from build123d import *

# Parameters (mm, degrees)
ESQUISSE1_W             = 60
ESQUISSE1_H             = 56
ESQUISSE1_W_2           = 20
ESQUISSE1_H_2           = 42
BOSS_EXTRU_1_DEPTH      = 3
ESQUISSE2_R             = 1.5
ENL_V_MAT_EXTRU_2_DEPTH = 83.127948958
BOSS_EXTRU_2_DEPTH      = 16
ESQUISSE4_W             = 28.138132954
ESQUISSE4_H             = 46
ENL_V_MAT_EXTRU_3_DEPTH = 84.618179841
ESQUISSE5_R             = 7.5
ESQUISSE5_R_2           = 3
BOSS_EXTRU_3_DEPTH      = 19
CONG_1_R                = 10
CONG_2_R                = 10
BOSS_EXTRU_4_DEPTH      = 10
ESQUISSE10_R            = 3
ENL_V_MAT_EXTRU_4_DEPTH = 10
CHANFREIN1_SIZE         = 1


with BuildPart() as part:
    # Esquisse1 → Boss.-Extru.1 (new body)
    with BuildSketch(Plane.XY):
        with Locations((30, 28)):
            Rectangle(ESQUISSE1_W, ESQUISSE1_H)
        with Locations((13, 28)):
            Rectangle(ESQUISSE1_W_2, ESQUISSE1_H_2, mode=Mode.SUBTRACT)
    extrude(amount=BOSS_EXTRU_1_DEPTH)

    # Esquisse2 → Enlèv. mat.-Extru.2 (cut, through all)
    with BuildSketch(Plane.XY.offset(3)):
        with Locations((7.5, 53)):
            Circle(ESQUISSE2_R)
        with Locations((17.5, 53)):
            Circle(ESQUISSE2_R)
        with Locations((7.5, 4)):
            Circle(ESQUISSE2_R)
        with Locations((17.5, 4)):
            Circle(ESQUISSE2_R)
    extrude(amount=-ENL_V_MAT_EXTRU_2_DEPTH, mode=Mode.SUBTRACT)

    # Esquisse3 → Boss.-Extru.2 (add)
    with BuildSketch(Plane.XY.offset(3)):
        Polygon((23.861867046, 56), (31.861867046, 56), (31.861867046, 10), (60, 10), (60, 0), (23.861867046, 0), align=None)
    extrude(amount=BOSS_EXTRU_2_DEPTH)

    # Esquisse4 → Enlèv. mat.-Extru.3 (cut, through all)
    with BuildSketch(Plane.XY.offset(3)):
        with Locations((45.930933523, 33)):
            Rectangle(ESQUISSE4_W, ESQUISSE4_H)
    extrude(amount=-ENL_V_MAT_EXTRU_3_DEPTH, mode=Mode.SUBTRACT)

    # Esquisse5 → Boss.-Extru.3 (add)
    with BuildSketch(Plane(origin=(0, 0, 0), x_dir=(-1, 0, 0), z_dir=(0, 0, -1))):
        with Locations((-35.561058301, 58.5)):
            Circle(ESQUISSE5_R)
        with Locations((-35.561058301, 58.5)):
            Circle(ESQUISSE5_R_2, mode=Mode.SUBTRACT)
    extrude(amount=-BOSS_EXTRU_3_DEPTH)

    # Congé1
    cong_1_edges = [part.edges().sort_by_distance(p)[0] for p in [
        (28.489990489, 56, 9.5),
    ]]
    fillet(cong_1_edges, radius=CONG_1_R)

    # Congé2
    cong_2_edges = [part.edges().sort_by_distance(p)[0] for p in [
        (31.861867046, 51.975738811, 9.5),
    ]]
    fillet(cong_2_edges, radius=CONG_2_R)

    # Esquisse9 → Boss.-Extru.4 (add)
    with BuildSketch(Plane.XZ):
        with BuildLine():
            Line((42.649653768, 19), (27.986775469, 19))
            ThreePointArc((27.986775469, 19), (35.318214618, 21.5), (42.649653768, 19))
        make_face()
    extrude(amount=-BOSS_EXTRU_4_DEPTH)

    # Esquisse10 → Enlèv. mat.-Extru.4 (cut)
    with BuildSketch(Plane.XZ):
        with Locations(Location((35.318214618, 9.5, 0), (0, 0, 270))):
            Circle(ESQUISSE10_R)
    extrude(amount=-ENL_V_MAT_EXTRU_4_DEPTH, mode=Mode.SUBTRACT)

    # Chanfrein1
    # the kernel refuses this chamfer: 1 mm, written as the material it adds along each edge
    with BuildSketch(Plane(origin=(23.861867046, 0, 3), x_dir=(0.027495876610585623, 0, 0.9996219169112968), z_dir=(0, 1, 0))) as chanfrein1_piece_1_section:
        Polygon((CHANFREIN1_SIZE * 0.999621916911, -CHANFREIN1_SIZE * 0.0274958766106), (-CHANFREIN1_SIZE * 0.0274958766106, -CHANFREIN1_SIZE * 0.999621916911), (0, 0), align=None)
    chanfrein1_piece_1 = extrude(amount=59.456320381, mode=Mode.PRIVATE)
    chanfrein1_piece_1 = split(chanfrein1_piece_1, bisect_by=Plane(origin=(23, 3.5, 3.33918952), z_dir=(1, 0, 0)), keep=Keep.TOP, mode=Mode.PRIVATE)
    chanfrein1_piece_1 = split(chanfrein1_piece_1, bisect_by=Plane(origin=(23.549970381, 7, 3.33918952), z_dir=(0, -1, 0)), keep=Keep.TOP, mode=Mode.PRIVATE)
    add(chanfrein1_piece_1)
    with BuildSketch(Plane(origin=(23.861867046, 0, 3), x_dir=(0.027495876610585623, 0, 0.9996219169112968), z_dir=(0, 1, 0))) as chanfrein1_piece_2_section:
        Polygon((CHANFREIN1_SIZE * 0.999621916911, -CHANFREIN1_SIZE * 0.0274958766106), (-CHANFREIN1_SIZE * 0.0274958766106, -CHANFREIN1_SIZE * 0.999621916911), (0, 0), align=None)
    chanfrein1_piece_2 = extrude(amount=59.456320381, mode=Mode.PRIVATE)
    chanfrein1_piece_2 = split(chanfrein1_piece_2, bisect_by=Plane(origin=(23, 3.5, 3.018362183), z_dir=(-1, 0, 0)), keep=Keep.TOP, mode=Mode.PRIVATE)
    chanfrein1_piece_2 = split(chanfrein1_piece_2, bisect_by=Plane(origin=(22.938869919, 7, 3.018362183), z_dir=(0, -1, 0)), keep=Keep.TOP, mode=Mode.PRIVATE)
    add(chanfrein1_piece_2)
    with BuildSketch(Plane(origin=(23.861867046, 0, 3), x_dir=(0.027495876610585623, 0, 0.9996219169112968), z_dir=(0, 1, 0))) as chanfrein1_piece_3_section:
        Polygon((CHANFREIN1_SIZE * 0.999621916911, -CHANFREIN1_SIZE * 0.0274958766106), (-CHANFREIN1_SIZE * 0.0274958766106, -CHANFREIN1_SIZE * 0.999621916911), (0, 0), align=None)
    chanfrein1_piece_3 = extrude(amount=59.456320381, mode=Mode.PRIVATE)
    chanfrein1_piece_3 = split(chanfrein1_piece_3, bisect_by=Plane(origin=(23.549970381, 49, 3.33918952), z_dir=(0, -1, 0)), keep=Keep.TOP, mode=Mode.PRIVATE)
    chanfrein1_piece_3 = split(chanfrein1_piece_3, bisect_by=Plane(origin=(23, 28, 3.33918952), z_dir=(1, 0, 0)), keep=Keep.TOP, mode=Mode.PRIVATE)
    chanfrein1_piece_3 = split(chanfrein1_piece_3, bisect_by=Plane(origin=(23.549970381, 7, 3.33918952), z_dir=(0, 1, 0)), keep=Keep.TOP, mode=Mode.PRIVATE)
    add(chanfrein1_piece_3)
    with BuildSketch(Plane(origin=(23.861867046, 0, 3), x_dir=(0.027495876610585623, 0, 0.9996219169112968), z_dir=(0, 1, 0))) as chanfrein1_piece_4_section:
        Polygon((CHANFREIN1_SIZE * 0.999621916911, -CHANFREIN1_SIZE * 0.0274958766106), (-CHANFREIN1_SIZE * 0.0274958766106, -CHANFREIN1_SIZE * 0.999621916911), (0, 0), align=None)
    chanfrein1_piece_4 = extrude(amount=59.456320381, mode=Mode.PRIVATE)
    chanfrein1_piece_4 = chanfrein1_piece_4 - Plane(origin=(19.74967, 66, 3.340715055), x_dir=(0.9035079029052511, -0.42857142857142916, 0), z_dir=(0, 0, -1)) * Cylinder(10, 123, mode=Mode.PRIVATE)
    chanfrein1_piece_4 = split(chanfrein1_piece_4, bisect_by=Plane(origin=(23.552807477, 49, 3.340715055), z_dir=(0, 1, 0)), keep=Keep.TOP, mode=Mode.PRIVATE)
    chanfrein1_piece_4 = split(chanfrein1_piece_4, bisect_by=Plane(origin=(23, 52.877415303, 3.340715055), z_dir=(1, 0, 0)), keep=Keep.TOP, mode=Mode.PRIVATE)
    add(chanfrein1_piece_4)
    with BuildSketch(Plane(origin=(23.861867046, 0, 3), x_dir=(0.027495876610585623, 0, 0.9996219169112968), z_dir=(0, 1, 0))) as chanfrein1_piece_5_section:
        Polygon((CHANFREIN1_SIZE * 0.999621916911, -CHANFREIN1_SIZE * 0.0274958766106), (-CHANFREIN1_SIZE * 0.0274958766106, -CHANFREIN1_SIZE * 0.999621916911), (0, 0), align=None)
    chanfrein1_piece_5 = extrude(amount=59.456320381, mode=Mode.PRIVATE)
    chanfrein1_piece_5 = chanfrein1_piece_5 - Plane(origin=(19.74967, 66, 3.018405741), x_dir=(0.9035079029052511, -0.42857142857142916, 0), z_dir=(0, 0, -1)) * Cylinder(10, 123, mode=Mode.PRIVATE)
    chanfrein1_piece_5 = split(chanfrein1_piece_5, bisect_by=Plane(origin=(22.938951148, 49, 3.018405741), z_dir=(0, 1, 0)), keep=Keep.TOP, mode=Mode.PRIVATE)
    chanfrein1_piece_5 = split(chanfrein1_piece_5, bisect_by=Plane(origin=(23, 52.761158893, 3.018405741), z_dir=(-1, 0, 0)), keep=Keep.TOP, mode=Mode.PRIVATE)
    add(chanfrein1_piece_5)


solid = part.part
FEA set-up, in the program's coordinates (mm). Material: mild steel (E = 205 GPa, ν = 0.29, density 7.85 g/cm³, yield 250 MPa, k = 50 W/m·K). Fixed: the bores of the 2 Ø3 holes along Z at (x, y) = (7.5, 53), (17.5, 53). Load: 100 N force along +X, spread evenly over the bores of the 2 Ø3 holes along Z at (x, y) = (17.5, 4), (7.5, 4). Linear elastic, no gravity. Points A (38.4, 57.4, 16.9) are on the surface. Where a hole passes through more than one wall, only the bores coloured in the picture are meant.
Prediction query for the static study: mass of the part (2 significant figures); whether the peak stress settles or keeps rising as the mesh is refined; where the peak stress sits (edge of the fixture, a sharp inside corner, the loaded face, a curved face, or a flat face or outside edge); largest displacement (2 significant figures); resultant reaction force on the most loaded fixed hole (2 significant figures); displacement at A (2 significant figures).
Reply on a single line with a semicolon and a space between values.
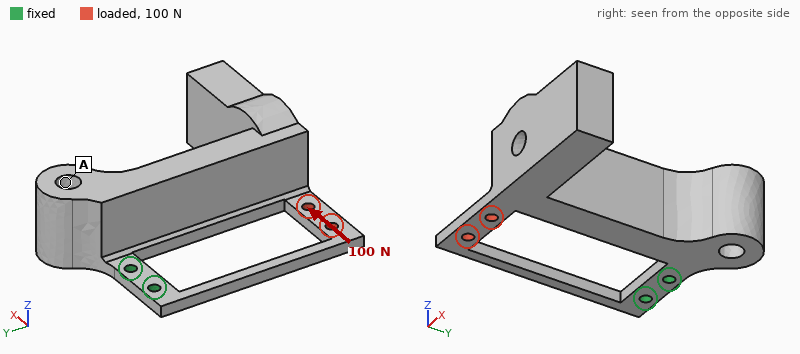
140 g; keeps rising; a sharp inside corner; 96 µm; 220 N; 23 µm
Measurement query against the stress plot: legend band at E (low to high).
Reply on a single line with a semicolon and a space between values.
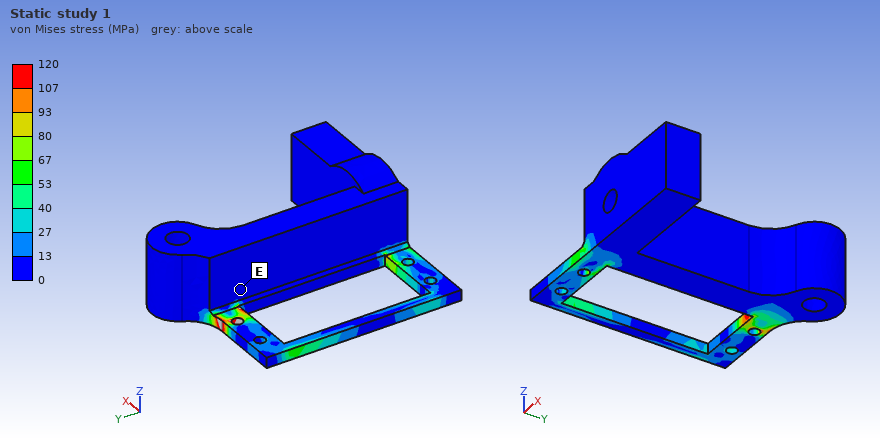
0 to 13 MPa
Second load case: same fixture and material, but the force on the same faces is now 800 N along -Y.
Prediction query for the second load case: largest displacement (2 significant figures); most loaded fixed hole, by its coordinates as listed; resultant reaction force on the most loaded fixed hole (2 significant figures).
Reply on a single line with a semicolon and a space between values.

22 µm; (17.5, 53); 430 N
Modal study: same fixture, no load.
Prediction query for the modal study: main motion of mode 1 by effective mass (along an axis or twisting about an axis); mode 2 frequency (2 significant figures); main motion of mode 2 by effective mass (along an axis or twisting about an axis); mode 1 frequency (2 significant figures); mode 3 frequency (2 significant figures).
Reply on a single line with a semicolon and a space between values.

along Z; 590 Hz; along X; 310 Hz; 920 Hz
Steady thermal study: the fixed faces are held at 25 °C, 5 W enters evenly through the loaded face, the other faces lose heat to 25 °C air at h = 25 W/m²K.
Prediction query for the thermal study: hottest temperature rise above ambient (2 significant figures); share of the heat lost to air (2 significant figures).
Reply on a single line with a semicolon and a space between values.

67 K; 65 %
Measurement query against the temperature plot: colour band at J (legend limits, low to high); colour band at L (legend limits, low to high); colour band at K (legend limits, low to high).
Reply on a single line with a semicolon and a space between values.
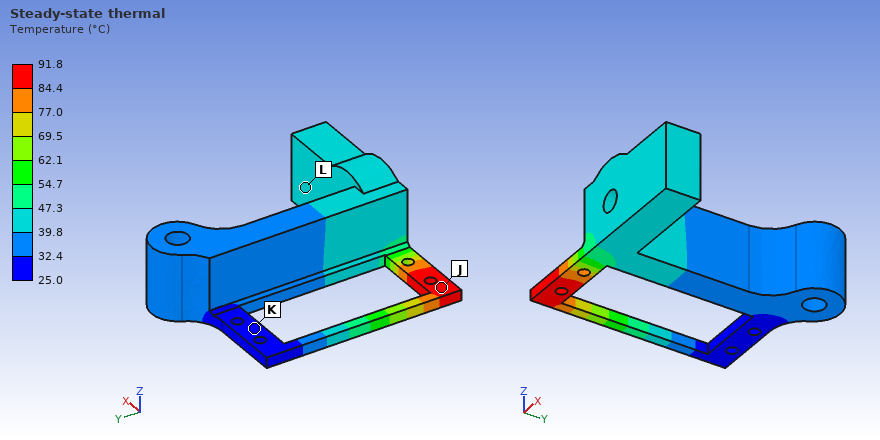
84.4 to 91.8 °C; 39.8 to 47.3 °C; 25.0 to 32.4 °C
